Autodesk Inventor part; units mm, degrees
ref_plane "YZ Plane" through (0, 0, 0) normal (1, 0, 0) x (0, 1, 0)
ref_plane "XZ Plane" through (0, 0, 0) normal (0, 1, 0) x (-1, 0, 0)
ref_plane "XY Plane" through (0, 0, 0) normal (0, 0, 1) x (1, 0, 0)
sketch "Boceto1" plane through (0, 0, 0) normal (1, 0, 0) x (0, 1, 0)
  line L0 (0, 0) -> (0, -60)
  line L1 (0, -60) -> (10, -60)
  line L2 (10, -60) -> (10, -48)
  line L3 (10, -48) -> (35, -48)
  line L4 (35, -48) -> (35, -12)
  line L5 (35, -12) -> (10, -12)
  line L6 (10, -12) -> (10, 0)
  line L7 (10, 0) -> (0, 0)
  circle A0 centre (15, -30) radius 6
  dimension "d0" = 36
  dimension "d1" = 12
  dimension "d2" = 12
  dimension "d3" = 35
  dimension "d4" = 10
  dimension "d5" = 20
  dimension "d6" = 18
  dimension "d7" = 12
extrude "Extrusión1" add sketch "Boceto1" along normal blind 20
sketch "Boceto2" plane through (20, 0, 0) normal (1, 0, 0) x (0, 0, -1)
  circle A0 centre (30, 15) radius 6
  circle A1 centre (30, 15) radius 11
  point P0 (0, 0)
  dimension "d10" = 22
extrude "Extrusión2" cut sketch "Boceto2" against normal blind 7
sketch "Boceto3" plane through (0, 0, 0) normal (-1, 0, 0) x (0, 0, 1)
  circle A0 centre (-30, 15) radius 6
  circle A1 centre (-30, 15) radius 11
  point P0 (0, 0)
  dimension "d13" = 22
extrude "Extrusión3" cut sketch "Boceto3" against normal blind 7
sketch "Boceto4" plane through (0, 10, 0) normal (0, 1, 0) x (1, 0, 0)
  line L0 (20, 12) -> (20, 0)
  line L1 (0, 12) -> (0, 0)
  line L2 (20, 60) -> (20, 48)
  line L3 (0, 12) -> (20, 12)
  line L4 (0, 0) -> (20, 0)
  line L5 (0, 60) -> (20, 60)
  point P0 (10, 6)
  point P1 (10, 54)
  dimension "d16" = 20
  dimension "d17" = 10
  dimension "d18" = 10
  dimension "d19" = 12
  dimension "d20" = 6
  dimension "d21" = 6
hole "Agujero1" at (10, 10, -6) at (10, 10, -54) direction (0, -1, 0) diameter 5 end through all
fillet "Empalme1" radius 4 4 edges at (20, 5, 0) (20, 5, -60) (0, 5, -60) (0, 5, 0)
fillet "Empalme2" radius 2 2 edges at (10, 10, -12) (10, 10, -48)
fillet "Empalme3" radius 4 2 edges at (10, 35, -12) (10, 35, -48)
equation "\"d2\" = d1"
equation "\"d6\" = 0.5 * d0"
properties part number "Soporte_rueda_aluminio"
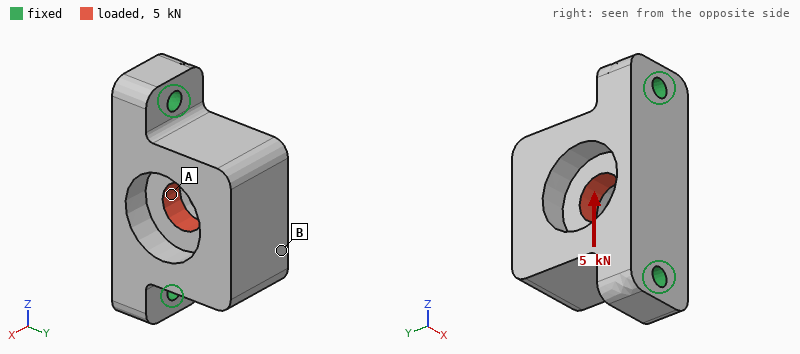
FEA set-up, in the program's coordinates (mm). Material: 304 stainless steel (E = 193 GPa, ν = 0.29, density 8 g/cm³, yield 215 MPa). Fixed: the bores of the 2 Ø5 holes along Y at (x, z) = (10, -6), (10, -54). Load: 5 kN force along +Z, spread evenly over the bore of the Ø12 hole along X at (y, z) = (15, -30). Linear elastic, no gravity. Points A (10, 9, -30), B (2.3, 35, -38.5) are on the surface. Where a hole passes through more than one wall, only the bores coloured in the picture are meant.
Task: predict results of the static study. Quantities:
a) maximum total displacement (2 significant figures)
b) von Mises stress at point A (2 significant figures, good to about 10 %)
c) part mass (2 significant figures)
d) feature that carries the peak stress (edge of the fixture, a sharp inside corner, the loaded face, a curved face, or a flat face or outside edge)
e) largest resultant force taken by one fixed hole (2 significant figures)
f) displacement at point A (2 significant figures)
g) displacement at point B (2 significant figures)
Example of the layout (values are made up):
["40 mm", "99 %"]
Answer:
["4.8 µm", "39 MPa", "190 g", "a curved face", "2.7 kN", "1.9 µm", "4.2 µm"]
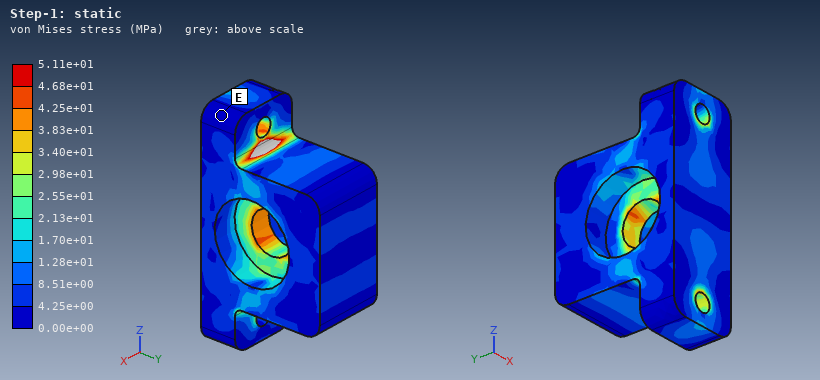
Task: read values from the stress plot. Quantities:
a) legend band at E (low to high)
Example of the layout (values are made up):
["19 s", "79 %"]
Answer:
["0.00e+00 to 4.25e+00 MPa"]
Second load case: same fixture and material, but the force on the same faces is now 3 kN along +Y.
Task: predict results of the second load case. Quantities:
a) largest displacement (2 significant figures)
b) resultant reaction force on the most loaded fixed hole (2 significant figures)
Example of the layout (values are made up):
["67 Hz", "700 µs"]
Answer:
["3.7 µm", "1.5 kN"]
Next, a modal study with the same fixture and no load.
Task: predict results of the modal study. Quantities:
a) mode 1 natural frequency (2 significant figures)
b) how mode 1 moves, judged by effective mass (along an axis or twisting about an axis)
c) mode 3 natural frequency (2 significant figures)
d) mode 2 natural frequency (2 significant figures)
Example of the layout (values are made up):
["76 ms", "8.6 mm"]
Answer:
["5600 Hz", "along X", "13 kHz", "13 kHz"]
